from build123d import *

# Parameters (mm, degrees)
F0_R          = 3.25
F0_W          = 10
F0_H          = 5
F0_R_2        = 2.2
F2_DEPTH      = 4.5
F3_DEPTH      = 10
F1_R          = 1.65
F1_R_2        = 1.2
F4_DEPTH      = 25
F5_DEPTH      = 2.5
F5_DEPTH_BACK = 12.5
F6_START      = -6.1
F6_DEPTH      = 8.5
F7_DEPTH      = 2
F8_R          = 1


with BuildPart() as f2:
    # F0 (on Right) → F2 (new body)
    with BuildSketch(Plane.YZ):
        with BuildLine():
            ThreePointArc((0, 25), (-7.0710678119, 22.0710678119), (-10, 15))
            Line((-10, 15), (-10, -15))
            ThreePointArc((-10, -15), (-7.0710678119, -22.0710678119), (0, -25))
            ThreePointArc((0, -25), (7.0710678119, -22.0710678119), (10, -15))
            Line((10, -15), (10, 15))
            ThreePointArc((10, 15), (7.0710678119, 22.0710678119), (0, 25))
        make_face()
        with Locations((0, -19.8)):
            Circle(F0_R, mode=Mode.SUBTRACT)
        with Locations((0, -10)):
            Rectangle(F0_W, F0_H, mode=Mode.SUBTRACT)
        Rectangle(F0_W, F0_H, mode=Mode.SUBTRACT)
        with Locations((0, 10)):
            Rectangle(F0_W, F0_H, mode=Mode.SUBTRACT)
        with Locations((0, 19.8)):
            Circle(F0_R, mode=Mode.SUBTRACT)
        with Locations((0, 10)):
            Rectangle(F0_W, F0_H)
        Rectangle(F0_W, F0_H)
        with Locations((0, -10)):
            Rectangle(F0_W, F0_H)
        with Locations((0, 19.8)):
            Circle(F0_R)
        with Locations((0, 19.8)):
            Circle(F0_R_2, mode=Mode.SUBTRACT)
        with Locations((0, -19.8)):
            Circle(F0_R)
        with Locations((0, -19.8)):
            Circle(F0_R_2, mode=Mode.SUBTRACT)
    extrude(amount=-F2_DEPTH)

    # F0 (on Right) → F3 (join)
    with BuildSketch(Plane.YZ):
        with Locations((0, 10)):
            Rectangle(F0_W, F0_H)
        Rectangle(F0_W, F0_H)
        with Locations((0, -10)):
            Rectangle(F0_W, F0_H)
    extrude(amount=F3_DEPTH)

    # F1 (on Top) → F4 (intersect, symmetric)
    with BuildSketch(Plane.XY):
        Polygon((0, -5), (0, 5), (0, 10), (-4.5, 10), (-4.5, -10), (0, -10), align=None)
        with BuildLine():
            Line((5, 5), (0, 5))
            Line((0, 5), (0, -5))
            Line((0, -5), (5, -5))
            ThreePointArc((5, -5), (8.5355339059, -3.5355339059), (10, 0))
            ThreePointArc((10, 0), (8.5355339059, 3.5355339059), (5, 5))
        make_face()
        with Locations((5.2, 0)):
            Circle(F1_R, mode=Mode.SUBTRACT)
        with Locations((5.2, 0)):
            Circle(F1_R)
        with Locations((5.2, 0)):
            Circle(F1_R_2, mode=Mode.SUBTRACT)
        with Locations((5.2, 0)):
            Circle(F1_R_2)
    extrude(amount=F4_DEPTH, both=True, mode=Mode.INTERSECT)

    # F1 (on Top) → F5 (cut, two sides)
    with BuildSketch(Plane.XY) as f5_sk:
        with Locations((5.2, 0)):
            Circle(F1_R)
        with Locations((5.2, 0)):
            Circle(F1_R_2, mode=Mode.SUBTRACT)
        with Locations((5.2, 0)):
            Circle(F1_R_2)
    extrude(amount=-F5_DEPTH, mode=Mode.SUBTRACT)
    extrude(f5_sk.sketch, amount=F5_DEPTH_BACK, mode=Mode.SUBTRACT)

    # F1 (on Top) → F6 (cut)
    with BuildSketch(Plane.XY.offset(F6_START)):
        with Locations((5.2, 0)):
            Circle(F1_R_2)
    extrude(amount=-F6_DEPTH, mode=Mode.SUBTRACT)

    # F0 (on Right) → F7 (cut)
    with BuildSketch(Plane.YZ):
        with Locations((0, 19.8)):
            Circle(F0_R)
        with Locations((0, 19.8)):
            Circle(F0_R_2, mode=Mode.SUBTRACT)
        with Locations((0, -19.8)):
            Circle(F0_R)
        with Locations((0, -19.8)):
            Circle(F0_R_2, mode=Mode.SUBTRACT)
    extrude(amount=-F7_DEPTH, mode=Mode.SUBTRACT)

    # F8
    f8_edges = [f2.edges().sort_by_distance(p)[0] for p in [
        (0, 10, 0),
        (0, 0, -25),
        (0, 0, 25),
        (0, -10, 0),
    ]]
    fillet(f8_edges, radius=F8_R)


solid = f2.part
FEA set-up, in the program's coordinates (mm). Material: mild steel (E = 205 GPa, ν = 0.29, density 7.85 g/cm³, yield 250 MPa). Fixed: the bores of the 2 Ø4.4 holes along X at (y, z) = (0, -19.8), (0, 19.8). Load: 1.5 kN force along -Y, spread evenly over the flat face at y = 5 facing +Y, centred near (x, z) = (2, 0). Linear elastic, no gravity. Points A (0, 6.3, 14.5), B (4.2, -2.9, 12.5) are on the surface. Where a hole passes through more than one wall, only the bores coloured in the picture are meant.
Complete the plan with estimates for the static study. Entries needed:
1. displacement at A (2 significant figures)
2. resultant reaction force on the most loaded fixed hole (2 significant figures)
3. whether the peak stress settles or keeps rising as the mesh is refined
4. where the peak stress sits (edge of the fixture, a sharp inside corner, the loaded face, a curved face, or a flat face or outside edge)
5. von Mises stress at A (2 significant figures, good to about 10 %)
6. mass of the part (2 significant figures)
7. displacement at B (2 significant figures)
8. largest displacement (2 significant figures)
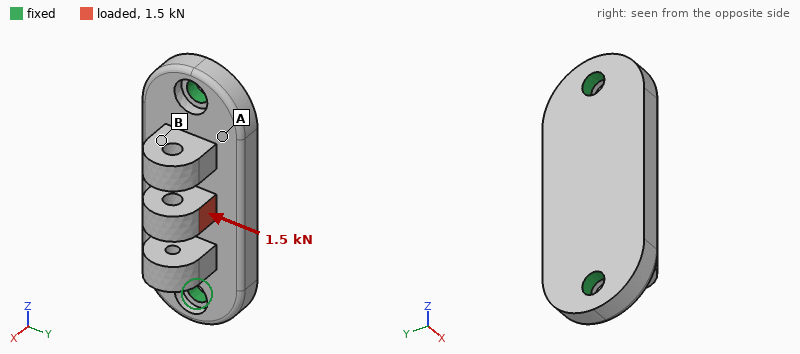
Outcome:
8.9 µm
750 N
keeps rising
edge of the fixture
35 MPa
40 g
13 µm
31 µm
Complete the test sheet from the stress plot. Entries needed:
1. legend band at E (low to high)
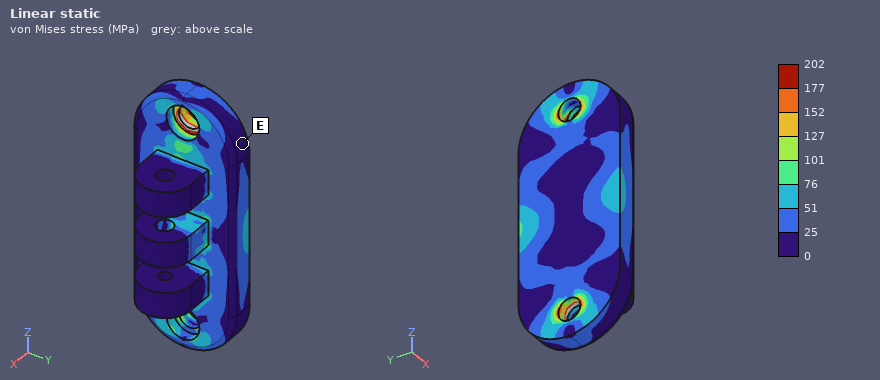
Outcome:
0 to 25 MPa
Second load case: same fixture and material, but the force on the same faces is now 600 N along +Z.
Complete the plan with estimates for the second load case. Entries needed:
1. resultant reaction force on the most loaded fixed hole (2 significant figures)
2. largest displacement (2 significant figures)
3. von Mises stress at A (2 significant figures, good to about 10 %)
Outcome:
330 N
6.1 µm
4.3 MPa
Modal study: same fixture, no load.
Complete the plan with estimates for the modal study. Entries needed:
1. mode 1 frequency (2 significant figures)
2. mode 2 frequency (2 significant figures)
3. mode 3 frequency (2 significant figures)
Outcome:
9300 Hz
9500 Hz
22 kHz
